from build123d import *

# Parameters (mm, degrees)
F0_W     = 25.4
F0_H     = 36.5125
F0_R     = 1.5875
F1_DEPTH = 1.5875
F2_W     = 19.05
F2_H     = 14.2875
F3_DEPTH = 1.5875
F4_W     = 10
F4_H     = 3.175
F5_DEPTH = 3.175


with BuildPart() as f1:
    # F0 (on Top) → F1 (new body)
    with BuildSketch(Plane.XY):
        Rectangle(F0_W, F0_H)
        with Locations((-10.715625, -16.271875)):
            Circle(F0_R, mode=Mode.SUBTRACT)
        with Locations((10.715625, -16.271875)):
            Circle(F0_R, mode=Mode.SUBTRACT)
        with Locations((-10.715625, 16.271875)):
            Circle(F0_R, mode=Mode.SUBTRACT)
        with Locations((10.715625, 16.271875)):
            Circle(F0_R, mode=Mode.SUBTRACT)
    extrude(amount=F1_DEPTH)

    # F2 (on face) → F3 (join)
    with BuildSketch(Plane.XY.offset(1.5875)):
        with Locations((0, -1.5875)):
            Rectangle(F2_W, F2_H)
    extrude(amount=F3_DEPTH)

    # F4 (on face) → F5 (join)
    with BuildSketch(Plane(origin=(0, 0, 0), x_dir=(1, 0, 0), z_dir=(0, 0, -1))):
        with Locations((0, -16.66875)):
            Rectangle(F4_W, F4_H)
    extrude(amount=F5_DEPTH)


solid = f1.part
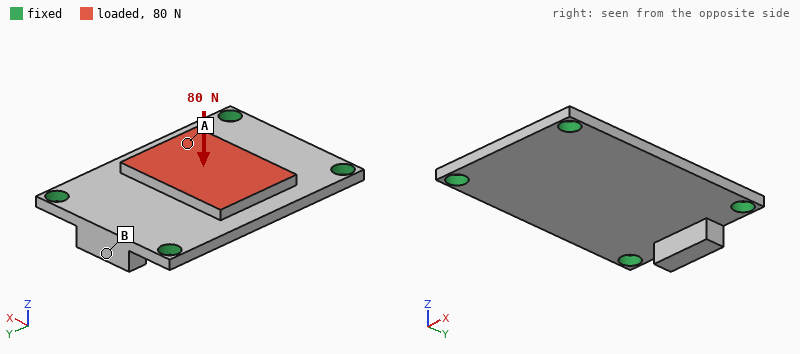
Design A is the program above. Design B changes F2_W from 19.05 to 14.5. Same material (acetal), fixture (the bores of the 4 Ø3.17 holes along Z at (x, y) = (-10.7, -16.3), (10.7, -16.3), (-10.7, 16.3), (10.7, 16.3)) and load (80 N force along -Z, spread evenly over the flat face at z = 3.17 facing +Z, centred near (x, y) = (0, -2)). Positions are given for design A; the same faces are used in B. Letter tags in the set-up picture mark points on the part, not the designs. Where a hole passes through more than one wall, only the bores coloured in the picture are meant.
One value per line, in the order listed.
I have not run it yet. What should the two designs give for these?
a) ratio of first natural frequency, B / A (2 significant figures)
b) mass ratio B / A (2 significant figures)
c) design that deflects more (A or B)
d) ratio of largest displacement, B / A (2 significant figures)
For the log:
0.98
0.95
B
1.2
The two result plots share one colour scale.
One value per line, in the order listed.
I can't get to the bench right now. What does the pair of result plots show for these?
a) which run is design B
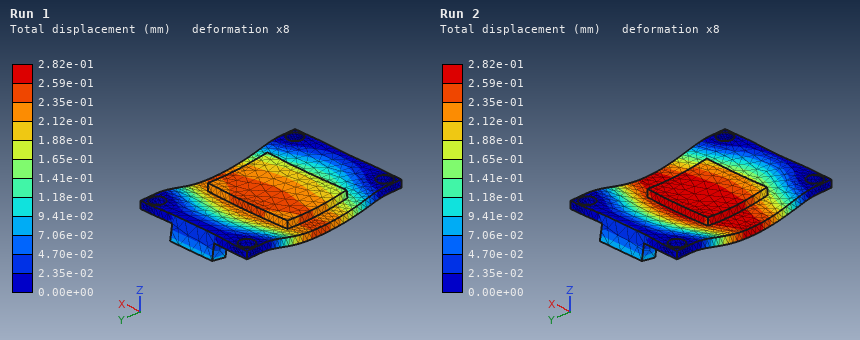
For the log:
Run 2
